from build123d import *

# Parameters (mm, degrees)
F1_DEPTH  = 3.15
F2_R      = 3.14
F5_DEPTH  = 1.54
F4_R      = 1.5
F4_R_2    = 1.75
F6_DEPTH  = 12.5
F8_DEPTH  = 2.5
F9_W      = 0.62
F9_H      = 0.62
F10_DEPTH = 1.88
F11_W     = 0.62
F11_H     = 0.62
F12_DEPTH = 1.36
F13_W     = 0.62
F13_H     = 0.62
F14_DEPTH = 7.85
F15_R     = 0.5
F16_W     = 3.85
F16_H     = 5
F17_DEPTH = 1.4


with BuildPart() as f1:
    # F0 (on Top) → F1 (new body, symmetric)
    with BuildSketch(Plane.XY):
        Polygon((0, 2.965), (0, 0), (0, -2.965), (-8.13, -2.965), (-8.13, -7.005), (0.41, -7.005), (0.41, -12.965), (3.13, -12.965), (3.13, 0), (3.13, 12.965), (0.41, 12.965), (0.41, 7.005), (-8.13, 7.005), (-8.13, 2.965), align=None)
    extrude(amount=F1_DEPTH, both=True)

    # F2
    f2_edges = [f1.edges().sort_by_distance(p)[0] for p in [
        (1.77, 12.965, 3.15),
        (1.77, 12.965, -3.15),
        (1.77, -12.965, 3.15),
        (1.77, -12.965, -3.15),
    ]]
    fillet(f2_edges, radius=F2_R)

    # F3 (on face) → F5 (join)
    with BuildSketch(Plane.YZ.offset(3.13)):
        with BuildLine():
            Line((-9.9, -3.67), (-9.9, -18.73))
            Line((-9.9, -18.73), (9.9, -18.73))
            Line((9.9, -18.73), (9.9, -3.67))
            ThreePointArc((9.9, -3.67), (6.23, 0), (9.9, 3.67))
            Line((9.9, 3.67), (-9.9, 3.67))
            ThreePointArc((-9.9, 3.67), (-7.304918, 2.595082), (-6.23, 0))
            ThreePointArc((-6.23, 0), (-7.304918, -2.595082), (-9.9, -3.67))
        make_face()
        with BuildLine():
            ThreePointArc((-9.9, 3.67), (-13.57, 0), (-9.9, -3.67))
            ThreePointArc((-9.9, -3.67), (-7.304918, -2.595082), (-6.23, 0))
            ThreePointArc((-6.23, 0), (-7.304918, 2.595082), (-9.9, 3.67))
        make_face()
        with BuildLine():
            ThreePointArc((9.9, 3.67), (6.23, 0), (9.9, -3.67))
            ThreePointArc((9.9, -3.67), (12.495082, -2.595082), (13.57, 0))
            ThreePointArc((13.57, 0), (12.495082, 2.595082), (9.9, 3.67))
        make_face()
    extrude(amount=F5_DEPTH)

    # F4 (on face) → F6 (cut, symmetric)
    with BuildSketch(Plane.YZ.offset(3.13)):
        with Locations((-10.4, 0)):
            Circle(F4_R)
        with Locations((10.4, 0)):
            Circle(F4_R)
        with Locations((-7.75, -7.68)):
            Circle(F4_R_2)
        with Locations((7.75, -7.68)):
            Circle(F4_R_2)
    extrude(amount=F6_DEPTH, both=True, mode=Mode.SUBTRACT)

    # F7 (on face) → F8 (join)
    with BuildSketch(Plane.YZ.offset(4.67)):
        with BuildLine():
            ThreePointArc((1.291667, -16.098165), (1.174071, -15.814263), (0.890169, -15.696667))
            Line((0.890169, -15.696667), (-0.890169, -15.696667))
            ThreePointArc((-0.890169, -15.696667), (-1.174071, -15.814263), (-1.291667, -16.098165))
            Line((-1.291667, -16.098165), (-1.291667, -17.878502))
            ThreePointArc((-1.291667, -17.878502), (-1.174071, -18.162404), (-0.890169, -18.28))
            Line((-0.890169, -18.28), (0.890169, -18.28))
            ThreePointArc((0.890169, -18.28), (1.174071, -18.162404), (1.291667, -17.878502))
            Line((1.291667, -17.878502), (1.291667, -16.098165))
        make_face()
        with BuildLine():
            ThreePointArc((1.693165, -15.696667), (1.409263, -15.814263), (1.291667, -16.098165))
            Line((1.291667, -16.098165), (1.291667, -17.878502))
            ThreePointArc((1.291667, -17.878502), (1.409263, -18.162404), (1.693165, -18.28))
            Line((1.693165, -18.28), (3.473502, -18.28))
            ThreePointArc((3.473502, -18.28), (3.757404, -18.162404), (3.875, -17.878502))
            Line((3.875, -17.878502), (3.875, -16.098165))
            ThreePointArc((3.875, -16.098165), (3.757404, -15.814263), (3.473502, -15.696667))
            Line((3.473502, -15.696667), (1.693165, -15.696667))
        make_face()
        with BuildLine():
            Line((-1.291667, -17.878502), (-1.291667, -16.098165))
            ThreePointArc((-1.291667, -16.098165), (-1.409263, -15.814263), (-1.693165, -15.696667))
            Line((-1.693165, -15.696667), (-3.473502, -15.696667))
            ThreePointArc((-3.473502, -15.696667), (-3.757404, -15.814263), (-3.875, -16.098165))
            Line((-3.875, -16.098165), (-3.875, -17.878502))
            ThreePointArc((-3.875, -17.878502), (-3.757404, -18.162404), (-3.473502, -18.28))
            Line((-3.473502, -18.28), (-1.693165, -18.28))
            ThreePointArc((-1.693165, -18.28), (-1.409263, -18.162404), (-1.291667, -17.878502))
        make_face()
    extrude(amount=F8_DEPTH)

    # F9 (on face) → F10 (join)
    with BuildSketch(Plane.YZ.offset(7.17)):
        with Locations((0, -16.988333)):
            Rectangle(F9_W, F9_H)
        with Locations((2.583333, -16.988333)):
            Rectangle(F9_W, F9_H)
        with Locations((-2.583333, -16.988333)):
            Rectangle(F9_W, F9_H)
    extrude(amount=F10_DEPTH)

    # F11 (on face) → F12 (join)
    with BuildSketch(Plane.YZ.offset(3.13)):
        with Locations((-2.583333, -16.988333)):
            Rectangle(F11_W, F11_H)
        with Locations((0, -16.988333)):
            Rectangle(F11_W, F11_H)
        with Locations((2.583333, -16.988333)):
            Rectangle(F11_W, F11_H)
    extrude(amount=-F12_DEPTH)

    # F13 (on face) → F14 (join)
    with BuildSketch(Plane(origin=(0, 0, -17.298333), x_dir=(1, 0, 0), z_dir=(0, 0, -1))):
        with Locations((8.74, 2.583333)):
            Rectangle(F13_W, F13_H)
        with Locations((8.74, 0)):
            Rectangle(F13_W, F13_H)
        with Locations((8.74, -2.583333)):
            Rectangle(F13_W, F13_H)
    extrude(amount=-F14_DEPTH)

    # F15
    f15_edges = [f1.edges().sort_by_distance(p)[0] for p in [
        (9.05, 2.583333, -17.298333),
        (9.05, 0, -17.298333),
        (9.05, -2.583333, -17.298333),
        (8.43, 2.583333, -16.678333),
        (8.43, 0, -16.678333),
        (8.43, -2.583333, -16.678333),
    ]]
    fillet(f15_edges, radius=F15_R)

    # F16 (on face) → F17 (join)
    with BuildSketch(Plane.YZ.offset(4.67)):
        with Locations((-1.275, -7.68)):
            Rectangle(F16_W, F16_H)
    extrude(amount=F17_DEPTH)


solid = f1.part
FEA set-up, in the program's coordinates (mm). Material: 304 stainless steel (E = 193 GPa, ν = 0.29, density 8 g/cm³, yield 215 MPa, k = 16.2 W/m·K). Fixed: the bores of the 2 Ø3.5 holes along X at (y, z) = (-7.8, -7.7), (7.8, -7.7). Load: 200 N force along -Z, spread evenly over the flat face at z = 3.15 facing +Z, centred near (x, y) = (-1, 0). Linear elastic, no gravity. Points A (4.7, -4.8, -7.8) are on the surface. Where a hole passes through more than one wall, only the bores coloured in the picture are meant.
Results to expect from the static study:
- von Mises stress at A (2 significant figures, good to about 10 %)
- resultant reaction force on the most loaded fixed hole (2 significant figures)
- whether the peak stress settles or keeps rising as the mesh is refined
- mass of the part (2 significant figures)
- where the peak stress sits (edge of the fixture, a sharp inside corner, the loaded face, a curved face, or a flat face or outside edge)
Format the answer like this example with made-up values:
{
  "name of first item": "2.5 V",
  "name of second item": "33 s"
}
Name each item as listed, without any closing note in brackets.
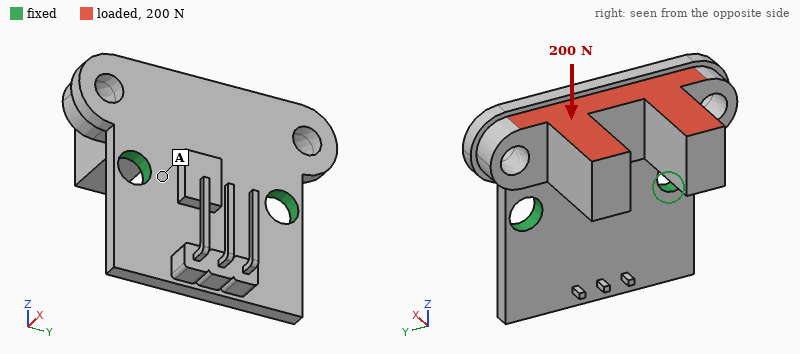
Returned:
{
  "von Mises stress at A": "24 MPa",
  "resultant reaction force on the most loaded fixed hole": "100 N",
  "whether the peak stress settles or keeps rising as the mesh is refined": "keeps rising",
  "mass of the part": "13 g",
  "where the peak stress sits": "edge of the fixture"
}
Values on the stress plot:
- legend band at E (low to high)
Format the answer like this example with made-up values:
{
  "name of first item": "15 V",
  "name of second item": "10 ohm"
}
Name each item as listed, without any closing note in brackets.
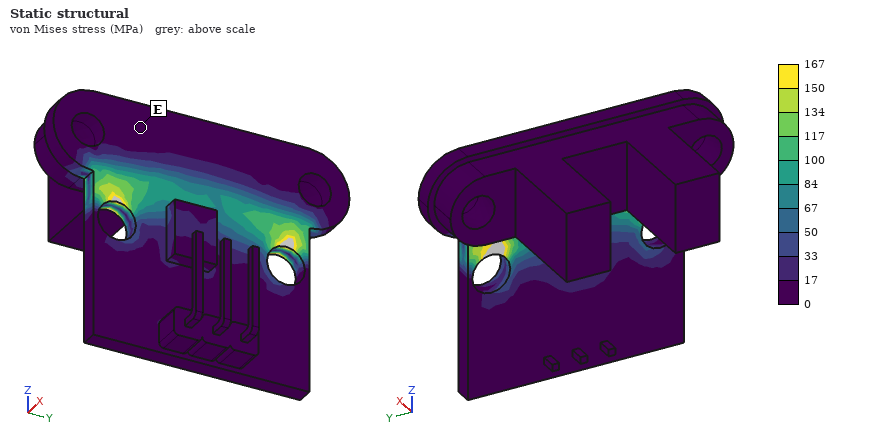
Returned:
{
  "legend band at E": "0 to 17 MPa"
}
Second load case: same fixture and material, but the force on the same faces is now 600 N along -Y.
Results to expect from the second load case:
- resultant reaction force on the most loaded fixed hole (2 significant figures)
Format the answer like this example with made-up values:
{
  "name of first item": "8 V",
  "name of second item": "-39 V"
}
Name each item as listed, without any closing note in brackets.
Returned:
{
  "resultant reaction force on the most loaded fixed hole": "520 N"
}
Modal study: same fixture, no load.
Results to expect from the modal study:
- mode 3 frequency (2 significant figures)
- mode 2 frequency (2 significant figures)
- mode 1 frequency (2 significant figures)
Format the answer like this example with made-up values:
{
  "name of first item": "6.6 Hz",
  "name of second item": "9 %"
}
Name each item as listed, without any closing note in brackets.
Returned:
{
  "mode 3 frequency": "6200 Hz",
  "mode 2 frequency": "6200 Hz",
  "mode 1 frequency": "3900 Hz"
}
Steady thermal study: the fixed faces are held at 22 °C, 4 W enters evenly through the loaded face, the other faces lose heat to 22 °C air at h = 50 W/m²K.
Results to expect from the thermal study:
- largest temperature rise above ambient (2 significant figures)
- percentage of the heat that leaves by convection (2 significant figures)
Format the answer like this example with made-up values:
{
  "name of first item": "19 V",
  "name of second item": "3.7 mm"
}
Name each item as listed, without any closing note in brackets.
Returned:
{
  "largest temperature rise above ambient": "46 K",
  "percentage of the heat that leaves by convection": "41 %"
}
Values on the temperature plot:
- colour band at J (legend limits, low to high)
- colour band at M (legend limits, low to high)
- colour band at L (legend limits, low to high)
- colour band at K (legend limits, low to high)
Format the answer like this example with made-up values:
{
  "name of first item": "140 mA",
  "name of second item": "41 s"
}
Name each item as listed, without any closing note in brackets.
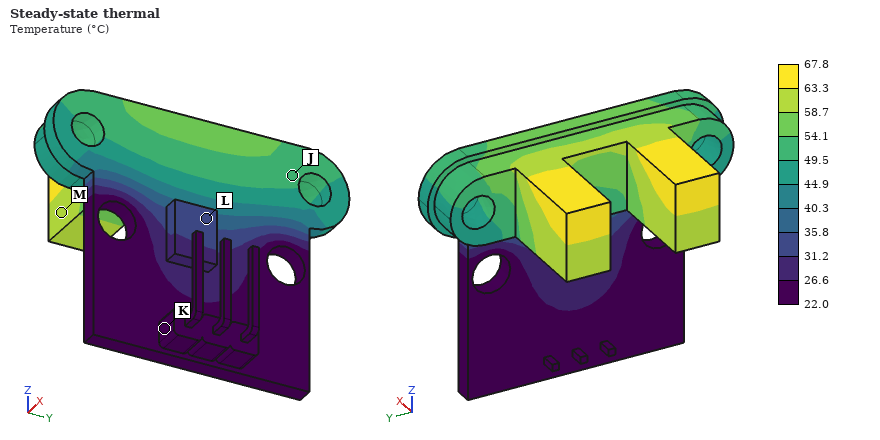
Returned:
{
  "colour band at J": "49.5 to 54.1 °C",
  "colour band at M": "58.7 to 63.3 °C",
  "colour band at L": "31.2 to 35.8 °C",
  "colour band at K": "22.0 to 26.6 °C"
}
